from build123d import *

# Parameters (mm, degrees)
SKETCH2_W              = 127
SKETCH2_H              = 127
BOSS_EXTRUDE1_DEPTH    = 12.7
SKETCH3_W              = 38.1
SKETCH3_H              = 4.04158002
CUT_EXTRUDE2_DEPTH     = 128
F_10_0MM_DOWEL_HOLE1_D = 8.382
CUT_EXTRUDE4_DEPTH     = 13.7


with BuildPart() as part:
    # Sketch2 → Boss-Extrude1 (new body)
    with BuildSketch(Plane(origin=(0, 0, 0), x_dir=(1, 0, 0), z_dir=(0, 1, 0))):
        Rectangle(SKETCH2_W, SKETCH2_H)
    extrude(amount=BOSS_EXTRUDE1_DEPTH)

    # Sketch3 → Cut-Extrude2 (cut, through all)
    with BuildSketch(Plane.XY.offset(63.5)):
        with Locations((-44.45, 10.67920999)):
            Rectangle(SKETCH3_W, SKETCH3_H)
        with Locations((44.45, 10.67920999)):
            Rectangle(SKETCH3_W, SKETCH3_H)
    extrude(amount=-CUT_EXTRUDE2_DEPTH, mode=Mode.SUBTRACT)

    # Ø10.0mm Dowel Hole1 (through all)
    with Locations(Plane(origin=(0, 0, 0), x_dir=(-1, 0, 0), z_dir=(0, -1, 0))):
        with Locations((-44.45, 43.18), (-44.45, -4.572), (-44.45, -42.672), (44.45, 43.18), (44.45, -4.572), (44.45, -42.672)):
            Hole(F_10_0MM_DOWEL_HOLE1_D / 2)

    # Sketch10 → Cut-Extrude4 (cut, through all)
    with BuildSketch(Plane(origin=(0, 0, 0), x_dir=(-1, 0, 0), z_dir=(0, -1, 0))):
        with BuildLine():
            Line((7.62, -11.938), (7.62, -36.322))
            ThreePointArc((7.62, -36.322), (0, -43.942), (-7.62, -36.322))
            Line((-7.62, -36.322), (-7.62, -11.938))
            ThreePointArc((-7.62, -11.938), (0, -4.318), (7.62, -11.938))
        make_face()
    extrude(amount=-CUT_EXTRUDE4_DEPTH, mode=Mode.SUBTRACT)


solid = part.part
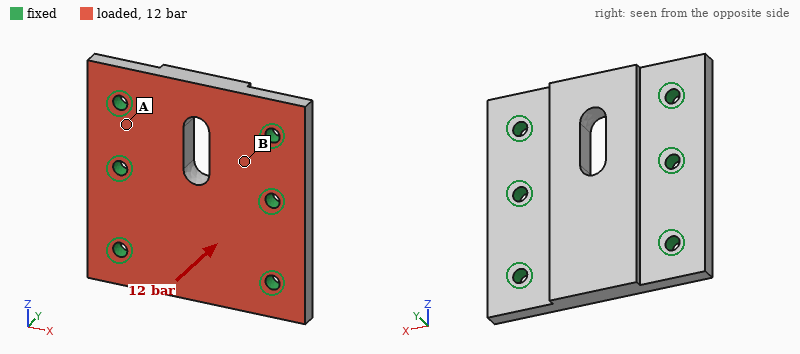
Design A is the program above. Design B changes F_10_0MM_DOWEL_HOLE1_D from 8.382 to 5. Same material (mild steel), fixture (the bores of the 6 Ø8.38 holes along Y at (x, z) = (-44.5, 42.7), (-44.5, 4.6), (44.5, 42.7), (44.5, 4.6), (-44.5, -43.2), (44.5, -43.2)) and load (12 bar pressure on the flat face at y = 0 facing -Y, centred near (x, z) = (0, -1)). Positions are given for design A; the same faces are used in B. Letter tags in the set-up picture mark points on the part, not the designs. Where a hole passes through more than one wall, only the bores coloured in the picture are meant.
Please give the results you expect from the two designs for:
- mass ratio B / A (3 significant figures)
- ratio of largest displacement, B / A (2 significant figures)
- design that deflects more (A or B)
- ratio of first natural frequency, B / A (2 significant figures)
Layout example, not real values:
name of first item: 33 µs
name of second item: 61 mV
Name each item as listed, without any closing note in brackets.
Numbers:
mass ratio B / A: 1.01
ratio of largest displacement, B / A: 1.3
design that deflects more: B
ratio of first natural frequency, B / A: 0.88
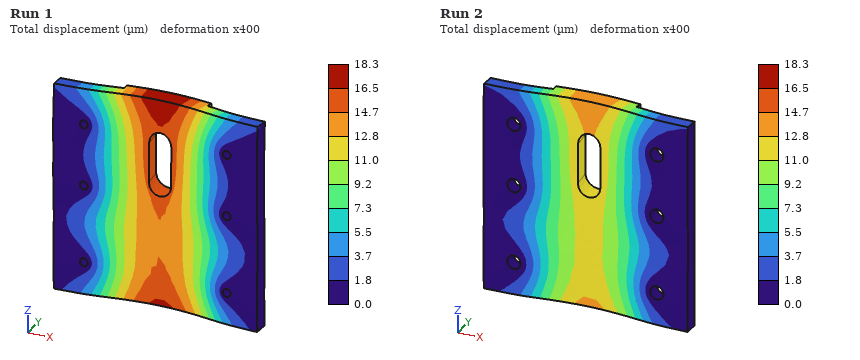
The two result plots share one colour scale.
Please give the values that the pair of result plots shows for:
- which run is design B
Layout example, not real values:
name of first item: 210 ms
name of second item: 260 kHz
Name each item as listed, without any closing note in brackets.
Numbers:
which run is design B: Run 1
